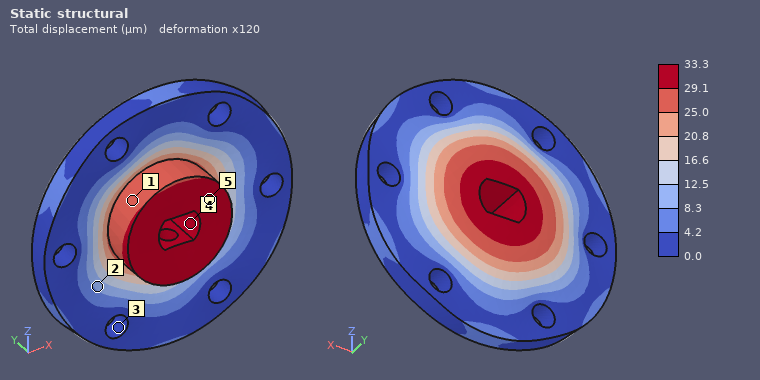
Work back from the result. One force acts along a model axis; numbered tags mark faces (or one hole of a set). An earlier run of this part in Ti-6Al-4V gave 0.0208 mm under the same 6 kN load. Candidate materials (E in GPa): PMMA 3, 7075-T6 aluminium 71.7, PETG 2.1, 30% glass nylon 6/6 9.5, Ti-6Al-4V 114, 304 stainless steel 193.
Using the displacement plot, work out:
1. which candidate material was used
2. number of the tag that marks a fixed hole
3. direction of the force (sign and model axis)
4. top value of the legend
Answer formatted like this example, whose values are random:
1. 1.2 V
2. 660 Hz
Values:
1. 7075-T6 aluminium
2. 3
3. +Y
4. 33.3 µm
